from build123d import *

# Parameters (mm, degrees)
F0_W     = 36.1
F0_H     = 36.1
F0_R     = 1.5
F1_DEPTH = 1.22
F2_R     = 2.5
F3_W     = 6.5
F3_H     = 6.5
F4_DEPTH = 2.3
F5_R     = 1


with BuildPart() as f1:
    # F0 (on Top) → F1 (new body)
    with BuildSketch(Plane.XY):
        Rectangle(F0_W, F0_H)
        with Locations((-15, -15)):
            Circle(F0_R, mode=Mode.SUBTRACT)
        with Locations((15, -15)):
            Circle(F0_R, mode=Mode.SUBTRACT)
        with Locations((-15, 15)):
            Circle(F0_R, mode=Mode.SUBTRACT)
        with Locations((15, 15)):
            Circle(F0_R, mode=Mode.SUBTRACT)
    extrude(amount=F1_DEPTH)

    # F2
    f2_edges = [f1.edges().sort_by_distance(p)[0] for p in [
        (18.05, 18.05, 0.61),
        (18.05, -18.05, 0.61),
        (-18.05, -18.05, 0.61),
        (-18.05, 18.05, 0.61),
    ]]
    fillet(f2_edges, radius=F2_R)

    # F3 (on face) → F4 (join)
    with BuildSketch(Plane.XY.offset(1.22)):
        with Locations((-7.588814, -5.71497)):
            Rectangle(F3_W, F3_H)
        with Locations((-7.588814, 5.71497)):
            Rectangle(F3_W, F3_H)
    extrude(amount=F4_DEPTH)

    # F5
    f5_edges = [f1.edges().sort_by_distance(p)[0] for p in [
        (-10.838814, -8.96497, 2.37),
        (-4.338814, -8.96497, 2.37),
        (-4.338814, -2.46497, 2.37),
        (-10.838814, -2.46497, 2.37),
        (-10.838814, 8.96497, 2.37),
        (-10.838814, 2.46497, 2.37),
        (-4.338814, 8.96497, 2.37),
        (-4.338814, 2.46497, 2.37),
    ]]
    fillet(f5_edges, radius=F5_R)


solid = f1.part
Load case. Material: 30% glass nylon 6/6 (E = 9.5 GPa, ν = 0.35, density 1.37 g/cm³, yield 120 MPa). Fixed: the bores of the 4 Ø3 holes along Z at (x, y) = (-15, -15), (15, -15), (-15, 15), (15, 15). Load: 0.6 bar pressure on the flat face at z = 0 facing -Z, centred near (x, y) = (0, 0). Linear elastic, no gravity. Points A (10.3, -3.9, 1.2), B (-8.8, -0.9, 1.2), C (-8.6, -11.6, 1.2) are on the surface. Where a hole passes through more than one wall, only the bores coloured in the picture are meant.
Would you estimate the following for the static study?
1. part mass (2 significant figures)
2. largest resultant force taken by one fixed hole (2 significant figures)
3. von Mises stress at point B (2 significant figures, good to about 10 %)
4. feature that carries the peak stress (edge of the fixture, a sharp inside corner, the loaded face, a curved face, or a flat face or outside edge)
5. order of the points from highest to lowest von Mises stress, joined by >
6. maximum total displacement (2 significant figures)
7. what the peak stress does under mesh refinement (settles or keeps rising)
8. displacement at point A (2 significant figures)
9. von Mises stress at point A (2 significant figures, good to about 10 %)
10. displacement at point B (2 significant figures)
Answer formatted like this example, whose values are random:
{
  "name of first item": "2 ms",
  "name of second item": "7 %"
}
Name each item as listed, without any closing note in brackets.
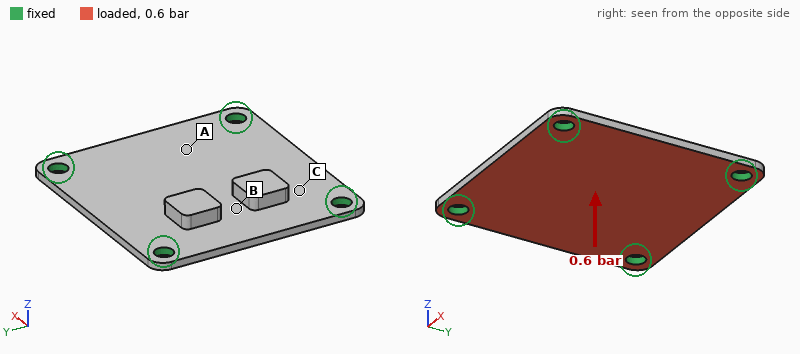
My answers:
{
  "part mass": "2.4 g",
  "largest resultant force taken by one fixed hole": "19 N",
  "von Mises stress at point B": "12 MPa",
  "feature that carries the peak stress": "edge of the fixture",
  "order of the points from highest to lowest von Mises stress, joined by >": "B > A > C",
  "maximum total displacement": "0.18 mm",
  "what the peak stress does under mesh refinement": "keeps rising",
  "displacement at point A": "0.12 mm",
  "von Mises stress at point A": "7.9 MPa",
  "displacement at point B": "0.13 mm"
}
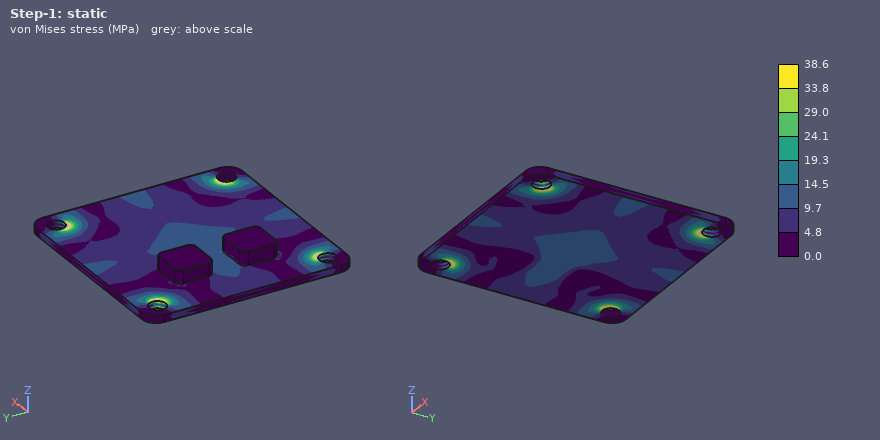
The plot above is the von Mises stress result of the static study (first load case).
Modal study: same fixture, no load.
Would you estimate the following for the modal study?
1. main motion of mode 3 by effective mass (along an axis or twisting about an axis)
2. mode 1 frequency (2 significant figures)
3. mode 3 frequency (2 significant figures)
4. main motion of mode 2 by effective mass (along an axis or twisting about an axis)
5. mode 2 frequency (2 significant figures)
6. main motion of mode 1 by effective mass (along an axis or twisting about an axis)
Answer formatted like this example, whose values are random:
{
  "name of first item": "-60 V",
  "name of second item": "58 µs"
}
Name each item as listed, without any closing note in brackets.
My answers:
{
  "main motion of mode 3 by effective mass": "twisting about X",
  "mode 1 frequency": "2600 Hz",
  "mode 3 frequency": "4700 Hz",
  "main motion of mode 2 by effective mass": "twisting about Y",
  "mode 2 frequency": "4500 Hz",
  "main motion of mode 1 by effective mass": "along Z"
}
